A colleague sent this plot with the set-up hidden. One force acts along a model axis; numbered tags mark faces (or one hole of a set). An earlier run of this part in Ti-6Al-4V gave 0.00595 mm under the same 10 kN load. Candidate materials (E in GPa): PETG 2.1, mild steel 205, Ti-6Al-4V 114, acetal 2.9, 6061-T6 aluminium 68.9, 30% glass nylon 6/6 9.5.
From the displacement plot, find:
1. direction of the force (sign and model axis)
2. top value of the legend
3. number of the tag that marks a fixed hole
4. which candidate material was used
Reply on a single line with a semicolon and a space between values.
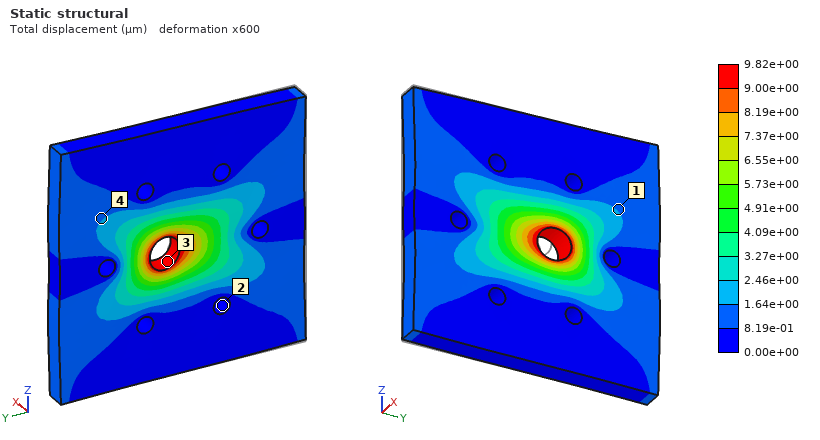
+Y; 9.82e+00 µm; 2; 6061-T6 aluminium
